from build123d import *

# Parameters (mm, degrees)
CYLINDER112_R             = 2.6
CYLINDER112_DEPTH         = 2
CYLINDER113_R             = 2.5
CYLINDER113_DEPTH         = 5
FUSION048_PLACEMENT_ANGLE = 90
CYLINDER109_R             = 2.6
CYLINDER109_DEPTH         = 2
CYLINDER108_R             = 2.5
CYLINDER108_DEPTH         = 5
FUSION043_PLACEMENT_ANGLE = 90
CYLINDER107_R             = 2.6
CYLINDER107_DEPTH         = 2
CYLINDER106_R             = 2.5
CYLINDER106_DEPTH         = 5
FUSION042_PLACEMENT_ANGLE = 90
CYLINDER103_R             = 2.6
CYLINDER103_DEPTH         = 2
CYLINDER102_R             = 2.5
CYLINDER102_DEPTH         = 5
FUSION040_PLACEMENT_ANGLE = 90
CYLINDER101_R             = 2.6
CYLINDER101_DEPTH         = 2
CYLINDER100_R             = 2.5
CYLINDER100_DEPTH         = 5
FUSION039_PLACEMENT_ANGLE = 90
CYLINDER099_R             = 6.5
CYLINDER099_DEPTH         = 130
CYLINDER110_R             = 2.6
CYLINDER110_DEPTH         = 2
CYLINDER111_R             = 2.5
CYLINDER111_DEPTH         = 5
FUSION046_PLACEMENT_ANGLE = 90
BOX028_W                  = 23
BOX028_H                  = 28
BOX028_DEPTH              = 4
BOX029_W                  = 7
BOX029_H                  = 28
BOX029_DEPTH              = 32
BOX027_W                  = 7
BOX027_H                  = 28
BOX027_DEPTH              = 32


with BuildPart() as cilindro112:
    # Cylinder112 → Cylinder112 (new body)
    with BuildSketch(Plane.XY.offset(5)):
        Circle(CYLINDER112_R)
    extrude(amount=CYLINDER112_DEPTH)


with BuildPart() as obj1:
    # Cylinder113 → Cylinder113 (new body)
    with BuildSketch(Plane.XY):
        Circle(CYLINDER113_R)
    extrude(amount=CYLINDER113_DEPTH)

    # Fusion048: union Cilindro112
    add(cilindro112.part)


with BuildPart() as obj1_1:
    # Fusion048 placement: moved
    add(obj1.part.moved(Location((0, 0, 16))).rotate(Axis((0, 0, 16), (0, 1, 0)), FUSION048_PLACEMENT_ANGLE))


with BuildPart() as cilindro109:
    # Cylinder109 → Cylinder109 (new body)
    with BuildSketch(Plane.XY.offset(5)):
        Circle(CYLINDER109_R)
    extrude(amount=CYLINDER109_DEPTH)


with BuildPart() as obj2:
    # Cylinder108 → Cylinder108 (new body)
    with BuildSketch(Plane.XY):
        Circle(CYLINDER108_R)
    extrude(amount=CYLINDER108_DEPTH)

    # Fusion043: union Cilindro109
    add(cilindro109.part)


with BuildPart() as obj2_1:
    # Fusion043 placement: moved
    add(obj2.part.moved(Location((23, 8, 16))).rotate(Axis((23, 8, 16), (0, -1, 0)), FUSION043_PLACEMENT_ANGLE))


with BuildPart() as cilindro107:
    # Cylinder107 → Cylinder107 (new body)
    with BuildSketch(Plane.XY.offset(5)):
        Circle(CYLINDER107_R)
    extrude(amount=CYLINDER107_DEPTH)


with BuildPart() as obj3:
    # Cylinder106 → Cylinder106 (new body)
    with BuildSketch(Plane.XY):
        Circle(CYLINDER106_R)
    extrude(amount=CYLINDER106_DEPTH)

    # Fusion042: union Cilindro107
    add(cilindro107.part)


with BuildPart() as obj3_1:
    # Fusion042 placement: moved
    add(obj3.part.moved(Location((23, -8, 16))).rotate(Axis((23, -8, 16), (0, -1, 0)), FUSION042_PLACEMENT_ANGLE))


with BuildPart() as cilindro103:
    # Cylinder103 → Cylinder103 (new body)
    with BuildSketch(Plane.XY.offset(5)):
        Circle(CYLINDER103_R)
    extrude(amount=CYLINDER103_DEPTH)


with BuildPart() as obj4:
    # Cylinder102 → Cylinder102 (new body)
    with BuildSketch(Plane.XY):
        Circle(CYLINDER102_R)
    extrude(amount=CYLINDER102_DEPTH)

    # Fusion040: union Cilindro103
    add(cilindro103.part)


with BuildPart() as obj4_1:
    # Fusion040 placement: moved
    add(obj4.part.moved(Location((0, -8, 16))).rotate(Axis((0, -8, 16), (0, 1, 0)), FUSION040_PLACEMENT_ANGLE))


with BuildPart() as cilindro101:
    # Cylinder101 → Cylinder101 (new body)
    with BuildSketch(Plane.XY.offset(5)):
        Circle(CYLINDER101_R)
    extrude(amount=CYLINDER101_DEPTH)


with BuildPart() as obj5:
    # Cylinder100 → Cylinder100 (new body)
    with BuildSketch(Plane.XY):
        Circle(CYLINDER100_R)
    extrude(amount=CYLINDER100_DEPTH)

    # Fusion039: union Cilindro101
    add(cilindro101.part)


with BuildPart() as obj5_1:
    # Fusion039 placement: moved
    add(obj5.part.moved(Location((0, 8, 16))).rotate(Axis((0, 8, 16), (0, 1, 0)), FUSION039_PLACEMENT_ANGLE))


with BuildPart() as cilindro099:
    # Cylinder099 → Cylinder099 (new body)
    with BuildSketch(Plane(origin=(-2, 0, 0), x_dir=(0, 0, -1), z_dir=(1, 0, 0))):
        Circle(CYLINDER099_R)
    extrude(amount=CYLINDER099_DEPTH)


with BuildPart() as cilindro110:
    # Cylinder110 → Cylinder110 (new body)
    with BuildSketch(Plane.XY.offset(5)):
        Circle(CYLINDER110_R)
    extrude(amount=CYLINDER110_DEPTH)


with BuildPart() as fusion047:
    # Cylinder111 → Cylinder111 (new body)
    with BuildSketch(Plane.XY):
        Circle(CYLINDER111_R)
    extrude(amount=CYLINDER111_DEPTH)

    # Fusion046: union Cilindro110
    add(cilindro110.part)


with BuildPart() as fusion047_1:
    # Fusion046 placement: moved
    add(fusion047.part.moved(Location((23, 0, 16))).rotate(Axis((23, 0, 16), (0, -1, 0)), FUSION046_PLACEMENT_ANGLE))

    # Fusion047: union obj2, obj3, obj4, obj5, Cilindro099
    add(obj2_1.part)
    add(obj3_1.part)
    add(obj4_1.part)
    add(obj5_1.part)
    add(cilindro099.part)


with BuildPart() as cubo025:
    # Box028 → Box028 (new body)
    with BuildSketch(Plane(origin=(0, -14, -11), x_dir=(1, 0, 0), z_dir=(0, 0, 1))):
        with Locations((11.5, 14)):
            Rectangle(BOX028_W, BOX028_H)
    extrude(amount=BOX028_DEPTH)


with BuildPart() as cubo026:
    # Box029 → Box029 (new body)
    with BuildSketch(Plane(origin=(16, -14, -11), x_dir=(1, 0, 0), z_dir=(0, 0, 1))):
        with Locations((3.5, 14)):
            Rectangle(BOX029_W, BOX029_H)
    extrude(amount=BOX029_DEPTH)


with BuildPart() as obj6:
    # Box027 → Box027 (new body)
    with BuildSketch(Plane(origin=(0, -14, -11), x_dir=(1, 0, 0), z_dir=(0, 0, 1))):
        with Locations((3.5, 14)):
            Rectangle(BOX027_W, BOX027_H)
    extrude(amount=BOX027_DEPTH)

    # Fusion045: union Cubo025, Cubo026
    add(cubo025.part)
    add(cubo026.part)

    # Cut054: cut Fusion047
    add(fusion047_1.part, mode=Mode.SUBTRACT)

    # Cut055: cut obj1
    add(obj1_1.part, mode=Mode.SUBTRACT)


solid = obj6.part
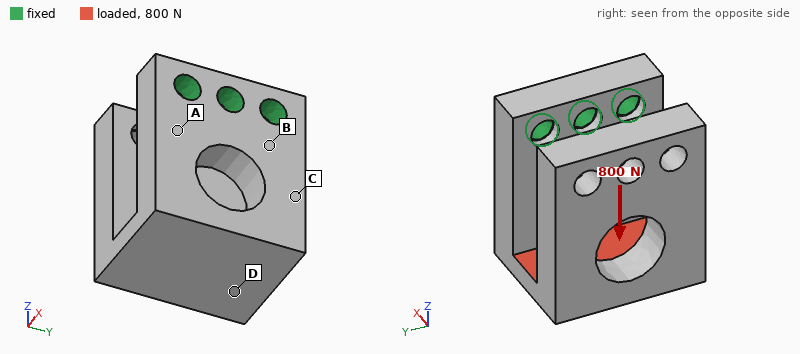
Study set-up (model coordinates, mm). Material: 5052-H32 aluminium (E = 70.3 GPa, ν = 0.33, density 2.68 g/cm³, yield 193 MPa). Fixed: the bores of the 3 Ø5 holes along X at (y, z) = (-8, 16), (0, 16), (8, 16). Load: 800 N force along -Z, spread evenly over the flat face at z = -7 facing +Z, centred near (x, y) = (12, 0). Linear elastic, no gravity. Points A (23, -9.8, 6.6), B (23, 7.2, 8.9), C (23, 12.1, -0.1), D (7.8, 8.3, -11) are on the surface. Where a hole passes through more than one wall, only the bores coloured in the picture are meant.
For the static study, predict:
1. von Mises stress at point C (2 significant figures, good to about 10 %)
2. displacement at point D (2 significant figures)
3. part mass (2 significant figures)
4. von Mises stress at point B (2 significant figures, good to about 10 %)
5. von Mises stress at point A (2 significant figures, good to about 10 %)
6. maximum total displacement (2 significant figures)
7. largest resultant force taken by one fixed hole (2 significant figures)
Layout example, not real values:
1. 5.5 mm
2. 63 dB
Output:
1. 44 MPa
2. 0.089 mm
3. 29 g
4. 28 MPa
5. 33 MPa
6. 0.17 mm
7. 370 N
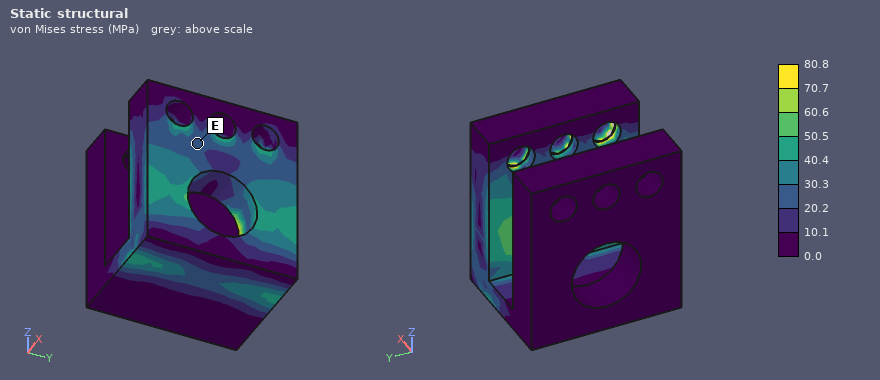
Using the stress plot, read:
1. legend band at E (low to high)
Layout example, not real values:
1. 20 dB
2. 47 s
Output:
1. 20.2 to 30.3 MPa
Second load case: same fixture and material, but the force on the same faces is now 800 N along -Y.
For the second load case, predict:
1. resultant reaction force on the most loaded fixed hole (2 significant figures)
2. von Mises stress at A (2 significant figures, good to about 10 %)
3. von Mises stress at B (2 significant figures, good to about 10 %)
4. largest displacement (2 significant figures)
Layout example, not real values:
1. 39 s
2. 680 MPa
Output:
1. 940 N
2. 31 MPa
3. 23 MPa
4. 90 µm
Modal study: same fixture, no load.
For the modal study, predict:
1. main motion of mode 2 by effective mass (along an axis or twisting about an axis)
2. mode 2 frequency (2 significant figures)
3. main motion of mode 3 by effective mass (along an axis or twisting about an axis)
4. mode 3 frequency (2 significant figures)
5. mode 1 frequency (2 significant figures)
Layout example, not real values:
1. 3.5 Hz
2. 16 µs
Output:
1. along Y
2. 2500 Hz
3. along X
4. 3300 Hz
5. 1700 Hz
